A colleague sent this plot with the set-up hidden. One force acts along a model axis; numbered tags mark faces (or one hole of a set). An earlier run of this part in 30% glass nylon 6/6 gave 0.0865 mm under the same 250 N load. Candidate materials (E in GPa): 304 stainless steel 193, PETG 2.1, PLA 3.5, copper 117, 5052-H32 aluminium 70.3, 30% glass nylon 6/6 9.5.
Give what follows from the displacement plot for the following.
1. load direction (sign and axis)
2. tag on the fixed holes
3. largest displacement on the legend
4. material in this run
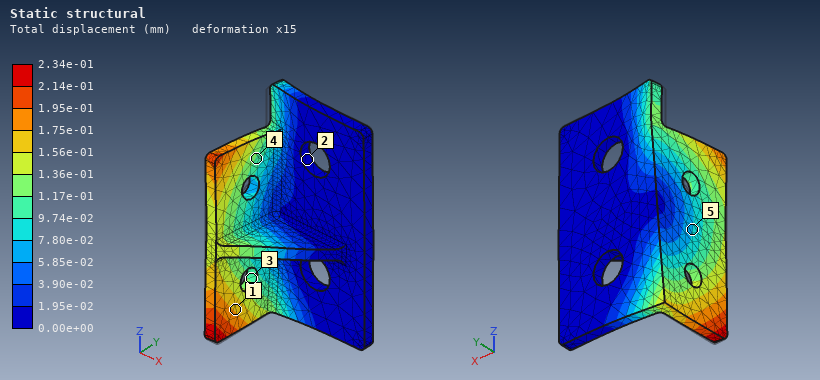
+Z
2
2.34e-01 mm
PLA
